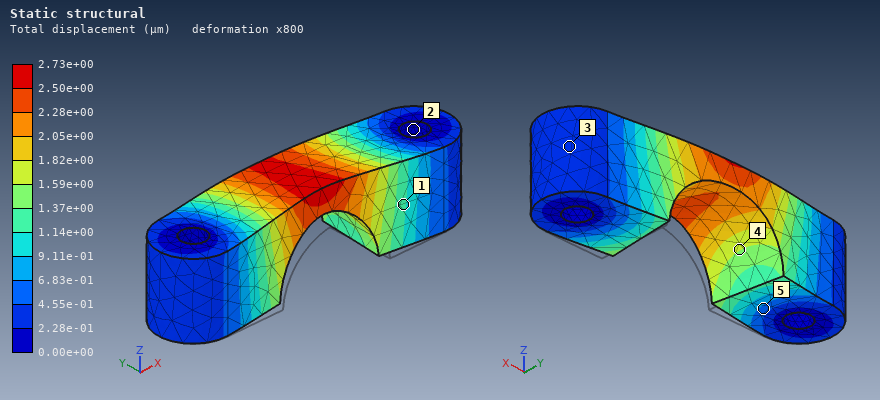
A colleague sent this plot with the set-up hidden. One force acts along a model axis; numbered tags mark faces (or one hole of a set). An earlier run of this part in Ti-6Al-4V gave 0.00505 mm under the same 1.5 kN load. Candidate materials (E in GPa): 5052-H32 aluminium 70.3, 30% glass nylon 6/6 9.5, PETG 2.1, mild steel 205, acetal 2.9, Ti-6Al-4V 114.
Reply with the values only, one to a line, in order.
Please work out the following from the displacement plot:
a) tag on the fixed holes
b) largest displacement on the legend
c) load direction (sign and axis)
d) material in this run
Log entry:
2
2.73e+00 µm
+Y
mild steel
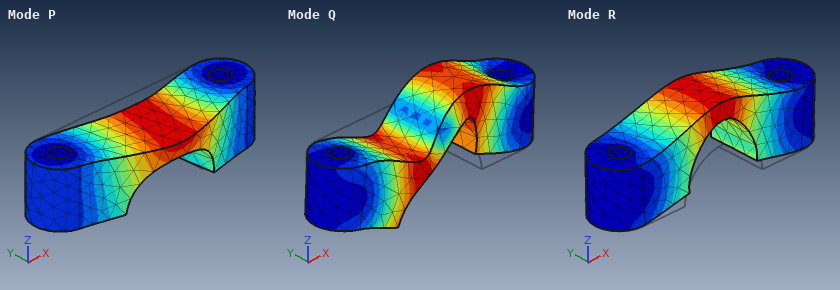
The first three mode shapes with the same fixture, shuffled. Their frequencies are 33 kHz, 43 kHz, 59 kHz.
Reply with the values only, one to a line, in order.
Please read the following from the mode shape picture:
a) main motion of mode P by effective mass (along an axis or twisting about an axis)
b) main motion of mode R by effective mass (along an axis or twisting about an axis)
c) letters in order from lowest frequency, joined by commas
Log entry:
along Y
along Z
P, R, Q
